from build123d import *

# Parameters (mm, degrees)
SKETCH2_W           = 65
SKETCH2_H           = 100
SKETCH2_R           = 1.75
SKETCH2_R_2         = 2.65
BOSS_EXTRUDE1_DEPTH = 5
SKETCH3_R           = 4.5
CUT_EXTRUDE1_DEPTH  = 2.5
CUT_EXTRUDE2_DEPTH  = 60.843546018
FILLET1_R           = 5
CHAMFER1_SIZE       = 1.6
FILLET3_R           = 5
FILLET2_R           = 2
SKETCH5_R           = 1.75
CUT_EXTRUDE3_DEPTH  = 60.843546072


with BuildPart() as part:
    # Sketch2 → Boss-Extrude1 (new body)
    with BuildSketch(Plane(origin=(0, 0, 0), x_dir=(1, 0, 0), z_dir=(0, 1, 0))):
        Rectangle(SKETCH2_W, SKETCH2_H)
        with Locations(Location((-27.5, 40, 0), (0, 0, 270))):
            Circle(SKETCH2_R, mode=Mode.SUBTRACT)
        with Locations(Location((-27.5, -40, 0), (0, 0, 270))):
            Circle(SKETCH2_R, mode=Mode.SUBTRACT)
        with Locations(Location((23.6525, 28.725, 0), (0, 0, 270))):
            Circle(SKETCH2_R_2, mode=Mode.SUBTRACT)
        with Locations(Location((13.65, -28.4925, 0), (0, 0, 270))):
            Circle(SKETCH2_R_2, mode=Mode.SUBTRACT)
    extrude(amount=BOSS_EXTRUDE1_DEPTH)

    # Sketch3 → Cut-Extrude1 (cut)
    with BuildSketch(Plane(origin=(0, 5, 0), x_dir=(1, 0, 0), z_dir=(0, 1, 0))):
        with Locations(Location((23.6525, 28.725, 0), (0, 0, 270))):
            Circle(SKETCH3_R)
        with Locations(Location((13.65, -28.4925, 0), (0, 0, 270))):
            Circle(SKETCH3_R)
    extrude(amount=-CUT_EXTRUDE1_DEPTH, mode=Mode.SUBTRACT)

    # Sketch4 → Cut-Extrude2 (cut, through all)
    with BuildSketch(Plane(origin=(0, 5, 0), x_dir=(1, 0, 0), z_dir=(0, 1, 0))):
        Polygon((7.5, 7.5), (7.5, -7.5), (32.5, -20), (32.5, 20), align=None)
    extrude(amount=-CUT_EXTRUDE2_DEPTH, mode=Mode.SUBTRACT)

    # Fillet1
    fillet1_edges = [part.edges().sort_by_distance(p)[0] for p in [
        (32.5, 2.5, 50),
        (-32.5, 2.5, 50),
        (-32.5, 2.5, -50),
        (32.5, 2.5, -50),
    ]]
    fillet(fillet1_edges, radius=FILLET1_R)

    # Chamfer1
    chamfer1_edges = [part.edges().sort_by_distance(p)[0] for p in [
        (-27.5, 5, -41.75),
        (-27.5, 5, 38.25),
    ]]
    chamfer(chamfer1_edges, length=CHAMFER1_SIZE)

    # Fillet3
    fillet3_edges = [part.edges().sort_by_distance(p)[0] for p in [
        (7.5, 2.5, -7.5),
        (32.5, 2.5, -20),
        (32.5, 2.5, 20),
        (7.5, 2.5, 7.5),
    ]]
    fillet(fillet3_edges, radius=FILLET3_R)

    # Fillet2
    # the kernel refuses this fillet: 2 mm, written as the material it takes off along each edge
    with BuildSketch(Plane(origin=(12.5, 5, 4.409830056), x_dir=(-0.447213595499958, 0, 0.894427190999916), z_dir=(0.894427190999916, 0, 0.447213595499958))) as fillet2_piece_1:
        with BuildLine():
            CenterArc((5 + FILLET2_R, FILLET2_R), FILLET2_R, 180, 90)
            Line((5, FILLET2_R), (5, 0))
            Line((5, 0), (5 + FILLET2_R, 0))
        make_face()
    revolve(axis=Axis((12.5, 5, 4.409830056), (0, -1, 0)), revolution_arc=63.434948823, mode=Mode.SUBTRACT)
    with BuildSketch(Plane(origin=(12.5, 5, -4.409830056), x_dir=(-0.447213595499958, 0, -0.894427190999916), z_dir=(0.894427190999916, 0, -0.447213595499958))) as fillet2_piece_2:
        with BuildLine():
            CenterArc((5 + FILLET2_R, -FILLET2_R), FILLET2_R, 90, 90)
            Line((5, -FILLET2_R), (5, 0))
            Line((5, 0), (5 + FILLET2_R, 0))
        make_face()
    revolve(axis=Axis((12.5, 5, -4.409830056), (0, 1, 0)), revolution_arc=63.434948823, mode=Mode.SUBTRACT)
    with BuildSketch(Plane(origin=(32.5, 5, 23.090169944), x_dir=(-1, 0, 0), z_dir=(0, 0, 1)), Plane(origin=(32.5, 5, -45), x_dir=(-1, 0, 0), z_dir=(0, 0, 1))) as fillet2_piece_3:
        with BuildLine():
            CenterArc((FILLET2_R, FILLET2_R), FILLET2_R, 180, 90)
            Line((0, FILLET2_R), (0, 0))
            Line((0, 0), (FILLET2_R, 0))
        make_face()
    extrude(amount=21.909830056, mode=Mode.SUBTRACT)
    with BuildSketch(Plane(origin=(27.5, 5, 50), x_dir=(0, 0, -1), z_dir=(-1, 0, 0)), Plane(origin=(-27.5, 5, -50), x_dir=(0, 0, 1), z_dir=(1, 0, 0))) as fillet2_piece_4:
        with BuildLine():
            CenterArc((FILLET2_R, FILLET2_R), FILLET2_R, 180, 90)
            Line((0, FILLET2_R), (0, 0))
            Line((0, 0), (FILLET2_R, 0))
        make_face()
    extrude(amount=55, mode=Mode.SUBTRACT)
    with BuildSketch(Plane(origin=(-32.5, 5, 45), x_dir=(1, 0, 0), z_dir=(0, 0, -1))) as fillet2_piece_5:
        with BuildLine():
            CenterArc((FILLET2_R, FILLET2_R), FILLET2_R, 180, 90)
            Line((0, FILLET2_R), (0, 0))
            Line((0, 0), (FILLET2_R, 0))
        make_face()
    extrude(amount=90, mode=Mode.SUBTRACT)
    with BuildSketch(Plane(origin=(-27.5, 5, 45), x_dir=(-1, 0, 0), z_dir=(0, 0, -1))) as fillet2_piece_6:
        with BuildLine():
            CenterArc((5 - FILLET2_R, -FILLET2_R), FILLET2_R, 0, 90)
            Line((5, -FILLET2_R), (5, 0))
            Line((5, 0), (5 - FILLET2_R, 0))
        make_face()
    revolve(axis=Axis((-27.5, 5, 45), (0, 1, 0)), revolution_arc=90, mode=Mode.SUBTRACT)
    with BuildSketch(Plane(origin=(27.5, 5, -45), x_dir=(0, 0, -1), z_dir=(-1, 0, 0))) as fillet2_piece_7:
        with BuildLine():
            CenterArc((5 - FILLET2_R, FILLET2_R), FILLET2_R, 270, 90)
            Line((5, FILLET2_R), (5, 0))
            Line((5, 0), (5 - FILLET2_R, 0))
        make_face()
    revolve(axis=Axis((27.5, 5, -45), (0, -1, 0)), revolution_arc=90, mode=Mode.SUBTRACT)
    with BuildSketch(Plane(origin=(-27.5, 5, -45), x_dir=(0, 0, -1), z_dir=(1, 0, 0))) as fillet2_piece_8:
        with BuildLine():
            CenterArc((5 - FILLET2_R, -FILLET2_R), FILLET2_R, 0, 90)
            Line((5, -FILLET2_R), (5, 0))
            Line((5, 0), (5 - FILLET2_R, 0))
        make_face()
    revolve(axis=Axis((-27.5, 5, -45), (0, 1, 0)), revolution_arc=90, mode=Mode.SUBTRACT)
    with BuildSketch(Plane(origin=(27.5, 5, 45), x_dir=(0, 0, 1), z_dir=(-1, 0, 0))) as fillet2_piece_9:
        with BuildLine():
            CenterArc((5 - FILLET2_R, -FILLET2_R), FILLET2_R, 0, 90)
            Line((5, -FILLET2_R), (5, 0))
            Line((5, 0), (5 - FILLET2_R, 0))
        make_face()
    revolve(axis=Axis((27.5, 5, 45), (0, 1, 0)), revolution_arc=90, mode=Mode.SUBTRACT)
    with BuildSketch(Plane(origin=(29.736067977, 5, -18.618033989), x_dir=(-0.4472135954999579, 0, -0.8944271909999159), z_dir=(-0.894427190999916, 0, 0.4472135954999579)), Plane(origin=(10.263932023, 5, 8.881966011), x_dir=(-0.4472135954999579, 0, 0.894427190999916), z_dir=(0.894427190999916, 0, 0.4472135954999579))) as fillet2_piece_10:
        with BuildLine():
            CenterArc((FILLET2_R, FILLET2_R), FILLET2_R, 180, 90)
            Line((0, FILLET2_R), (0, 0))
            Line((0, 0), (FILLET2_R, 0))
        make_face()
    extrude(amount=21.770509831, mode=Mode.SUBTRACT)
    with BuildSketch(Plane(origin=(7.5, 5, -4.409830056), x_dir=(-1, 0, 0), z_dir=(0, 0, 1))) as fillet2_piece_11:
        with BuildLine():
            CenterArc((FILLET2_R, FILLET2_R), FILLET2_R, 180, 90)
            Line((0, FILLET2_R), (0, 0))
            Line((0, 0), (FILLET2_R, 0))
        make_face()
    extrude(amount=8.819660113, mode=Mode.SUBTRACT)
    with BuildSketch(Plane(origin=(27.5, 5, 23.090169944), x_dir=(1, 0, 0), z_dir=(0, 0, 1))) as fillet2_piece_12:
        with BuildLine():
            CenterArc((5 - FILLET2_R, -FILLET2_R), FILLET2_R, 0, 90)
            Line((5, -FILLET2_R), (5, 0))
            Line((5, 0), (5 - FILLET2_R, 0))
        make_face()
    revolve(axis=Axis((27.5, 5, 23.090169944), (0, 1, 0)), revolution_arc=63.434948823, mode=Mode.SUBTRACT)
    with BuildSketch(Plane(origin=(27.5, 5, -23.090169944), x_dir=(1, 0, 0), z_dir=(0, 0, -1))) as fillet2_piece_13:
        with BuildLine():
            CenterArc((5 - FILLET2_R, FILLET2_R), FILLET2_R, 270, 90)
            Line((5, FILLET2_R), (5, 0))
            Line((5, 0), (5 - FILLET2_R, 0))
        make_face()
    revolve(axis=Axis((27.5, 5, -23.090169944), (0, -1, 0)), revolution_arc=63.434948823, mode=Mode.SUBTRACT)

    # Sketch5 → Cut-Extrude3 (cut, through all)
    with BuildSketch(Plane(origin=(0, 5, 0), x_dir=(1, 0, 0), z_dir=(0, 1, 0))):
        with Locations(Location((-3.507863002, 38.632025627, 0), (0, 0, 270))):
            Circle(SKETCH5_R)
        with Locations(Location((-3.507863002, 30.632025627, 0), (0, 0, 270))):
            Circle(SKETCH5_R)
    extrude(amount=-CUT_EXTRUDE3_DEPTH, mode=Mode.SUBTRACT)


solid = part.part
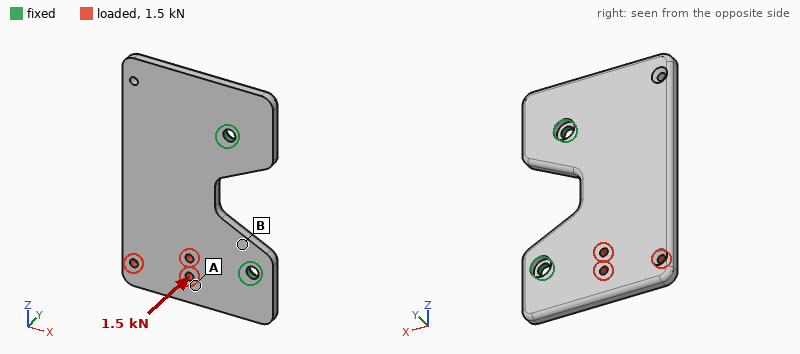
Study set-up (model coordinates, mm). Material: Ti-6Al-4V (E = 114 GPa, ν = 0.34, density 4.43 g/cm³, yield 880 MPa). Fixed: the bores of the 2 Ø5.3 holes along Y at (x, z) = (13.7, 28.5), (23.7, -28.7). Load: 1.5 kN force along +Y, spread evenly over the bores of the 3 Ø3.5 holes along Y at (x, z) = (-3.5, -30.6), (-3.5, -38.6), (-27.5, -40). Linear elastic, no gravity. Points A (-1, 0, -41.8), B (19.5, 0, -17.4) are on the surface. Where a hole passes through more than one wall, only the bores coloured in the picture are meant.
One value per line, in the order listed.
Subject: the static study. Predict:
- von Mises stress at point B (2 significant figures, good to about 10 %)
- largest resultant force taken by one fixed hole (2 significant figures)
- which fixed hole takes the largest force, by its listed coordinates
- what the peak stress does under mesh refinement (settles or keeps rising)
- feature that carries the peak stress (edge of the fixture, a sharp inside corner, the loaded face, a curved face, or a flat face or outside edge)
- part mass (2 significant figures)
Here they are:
160 MPa
1.4 kN
(23.7, -28.7)
keeps rising
edge of the fixture
120 g
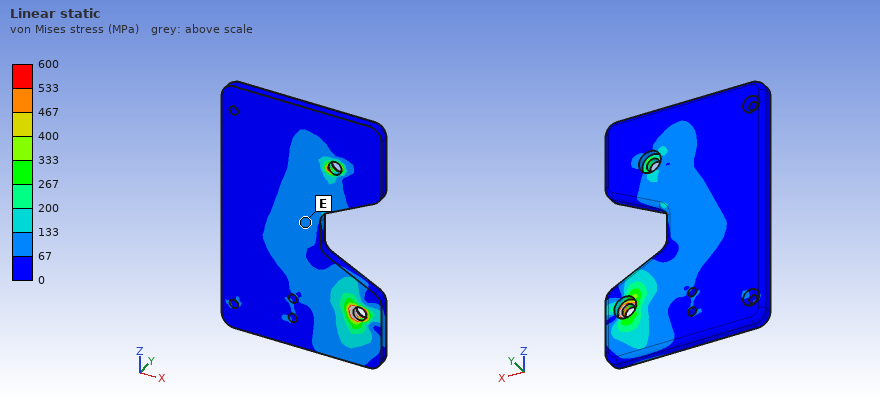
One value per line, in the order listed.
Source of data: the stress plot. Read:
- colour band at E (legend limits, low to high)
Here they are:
67 to 133 MPa
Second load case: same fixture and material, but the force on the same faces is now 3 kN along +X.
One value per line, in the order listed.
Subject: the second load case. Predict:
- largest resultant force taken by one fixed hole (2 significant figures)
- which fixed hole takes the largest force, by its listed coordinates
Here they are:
3.3 kN
(23.7, -28.7)
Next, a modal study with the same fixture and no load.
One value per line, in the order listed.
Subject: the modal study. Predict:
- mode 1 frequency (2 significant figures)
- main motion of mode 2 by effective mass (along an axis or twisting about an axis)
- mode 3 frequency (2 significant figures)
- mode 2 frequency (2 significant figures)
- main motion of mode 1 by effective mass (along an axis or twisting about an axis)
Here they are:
1000 Hz
twisting about X
3500 Hz
1900 Hz
along Y
